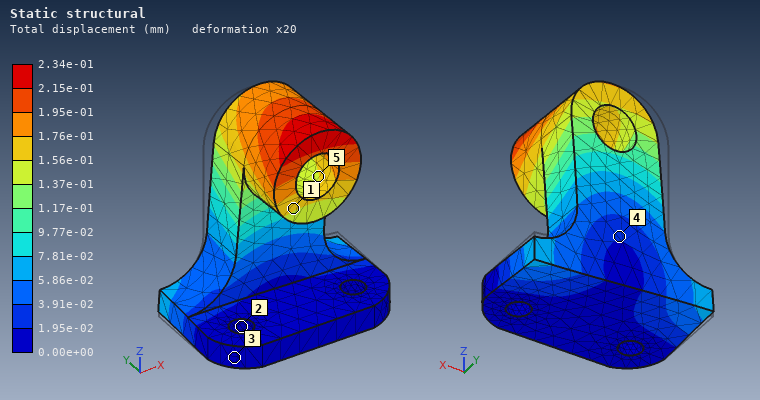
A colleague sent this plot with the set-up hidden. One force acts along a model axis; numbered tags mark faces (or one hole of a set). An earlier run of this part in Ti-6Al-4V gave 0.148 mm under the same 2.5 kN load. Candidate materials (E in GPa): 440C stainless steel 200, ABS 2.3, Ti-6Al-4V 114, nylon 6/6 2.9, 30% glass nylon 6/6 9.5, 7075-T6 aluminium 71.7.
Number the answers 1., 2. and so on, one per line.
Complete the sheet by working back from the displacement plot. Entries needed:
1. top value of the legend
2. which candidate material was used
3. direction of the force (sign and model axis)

1. 2.34e-01 mm
2. 7075-T6 aluminium
3. +X
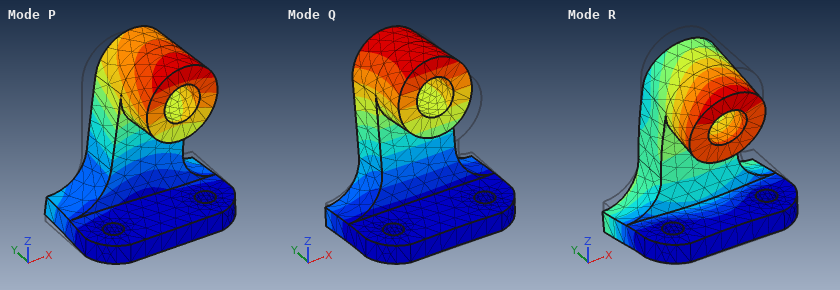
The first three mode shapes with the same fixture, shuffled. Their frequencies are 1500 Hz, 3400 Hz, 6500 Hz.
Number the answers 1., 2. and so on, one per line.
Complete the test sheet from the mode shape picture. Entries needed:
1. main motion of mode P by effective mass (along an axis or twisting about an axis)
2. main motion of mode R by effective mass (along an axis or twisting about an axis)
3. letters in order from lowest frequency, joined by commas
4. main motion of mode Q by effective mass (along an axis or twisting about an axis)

1. along X
2. along Z
3. Q, P, R
4. along Y
